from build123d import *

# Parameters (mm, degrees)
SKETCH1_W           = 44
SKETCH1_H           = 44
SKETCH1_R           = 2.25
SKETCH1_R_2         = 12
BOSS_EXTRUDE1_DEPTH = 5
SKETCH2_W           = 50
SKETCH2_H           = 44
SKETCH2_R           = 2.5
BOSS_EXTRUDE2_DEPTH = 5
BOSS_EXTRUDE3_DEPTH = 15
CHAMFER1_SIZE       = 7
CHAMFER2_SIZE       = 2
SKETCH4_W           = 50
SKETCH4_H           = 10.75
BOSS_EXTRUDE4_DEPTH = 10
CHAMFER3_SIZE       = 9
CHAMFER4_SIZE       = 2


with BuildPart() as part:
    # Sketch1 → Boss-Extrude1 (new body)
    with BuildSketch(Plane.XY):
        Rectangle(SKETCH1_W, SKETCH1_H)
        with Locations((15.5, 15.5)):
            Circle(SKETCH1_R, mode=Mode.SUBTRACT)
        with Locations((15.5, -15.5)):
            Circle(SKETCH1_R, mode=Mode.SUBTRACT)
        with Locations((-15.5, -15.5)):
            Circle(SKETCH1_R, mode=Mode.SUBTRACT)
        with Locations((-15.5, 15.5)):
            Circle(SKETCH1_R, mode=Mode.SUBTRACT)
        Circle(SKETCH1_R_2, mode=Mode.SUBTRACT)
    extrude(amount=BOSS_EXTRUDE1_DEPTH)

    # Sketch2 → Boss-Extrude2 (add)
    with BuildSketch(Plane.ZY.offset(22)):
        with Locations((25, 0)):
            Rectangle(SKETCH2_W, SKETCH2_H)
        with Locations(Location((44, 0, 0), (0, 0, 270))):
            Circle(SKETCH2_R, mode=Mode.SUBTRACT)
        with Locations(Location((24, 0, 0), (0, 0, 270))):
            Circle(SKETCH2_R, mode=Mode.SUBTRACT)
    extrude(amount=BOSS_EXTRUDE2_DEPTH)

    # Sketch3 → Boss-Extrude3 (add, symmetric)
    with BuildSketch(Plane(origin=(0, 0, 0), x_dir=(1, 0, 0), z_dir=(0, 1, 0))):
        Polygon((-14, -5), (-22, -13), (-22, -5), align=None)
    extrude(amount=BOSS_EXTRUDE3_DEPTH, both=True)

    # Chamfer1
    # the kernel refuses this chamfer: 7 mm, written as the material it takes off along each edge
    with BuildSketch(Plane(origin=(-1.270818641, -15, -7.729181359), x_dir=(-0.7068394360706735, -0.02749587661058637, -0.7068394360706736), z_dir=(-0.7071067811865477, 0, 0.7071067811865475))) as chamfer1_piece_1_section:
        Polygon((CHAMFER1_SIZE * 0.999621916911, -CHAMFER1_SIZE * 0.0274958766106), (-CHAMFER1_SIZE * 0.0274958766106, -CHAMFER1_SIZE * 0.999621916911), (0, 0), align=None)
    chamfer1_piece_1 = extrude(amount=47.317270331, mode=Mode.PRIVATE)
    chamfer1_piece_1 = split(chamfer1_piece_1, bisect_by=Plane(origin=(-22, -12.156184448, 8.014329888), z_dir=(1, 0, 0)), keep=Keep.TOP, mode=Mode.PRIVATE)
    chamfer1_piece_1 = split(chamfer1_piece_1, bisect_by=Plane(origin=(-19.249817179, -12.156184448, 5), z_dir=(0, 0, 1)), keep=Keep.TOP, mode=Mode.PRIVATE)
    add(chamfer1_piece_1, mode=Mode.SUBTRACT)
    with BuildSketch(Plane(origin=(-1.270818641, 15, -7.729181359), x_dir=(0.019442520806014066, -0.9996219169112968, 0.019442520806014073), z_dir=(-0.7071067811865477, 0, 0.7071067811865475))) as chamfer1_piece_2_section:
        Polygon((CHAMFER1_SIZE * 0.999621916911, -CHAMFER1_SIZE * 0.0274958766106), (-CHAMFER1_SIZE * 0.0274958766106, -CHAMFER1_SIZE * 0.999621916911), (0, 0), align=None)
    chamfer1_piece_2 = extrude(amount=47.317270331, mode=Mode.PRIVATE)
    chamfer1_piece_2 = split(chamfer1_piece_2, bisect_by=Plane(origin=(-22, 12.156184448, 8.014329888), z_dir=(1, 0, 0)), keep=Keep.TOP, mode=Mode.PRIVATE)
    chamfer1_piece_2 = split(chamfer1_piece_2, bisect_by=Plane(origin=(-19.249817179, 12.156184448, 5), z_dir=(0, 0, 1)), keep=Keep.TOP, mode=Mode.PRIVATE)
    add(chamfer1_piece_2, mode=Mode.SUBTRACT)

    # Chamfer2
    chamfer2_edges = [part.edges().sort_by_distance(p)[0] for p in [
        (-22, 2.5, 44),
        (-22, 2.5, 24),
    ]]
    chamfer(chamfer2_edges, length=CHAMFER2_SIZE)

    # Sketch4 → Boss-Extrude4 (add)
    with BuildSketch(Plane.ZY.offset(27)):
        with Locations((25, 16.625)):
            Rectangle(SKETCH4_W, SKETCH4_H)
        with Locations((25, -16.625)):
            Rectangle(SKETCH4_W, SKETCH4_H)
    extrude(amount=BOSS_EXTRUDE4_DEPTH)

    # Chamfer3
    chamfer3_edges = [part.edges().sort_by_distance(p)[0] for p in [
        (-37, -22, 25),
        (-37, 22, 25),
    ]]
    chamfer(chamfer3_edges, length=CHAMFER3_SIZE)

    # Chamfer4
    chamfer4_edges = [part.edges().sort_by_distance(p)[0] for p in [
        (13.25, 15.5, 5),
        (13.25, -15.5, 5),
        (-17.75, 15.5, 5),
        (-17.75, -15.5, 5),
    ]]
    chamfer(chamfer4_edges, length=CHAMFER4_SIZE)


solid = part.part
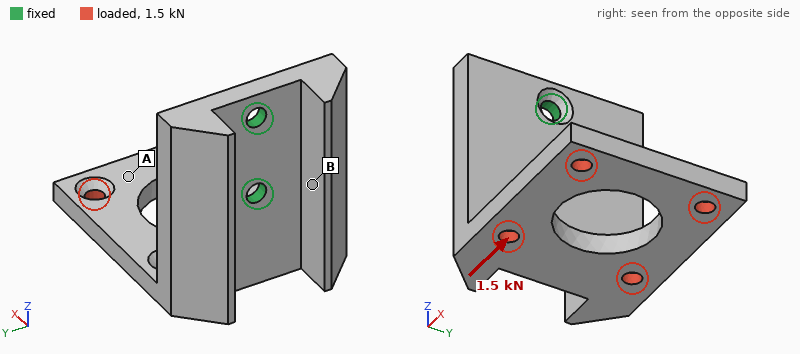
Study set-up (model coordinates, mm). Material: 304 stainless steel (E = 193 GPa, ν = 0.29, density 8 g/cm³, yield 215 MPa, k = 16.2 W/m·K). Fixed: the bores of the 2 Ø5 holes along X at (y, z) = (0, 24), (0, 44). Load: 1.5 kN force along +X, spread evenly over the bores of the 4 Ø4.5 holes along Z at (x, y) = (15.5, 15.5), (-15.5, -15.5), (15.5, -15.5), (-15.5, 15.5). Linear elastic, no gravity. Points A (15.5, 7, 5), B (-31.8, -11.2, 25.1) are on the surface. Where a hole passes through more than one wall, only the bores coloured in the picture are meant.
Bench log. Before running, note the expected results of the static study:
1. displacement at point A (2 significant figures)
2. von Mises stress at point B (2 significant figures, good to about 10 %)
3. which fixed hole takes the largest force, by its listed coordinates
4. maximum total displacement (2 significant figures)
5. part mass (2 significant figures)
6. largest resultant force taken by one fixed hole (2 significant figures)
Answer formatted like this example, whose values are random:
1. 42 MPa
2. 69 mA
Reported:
1. 0.091 mm
2. 24 MPa
3. (0, 24)
4. 0.11 mm
5. 200 g
6. 2.7 kN
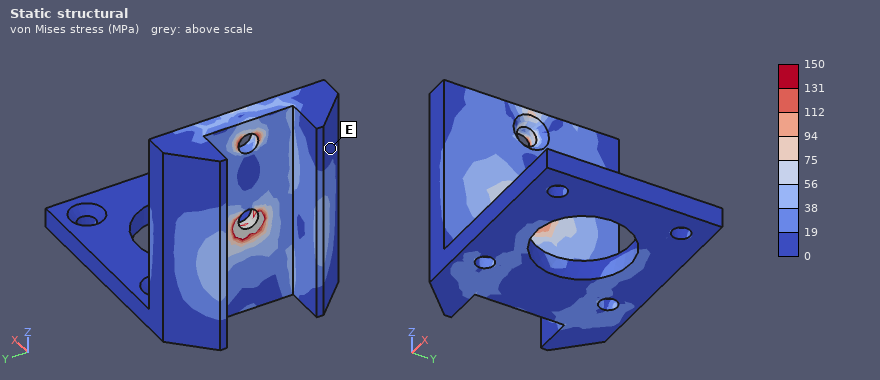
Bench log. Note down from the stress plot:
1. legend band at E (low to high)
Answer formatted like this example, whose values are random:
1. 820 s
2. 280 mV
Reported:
1. 0 to 19 MPa
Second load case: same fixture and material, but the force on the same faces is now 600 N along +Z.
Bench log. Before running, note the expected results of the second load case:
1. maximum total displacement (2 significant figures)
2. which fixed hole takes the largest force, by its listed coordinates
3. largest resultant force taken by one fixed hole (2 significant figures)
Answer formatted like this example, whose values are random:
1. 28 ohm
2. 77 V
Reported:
1. 0.17 mm
2. (0, 24)
3. 790 N
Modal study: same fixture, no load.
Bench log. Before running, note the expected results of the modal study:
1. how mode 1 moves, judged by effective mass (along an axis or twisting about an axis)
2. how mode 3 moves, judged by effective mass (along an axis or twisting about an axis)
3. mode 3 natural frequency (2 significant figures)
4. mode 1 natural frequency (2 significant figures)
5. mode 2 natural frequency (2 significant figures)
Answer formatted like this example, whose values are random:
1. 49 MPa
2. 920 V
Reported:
1. along Z
2. along X
3. 3600 Hz
4. 1500 Hz
5. 1700 Hz
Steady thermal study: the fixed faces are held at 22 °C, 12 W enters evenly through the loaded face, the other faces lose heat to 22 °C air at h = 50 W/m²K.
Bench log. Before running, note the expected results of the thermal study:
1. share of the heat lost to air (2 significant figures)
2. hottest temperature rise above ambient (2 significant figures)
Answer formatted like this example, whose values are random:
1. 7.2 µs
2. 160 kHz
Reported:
1. 81 %
2. 60 K
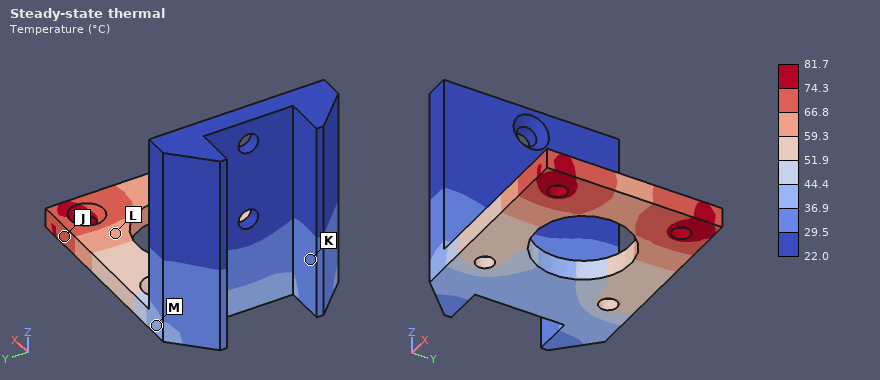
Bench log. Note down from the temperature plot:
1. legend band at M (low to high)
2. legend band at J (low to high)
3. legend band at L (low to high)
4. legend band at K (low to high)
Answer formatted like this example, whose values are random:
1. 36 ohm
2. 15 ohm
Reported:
1. 36.9 to 44.4 °C
2. 66.8 to 74.3 °C
3. 59.3 to 66.8 °C
4. 29.5 to 36.9 °C
